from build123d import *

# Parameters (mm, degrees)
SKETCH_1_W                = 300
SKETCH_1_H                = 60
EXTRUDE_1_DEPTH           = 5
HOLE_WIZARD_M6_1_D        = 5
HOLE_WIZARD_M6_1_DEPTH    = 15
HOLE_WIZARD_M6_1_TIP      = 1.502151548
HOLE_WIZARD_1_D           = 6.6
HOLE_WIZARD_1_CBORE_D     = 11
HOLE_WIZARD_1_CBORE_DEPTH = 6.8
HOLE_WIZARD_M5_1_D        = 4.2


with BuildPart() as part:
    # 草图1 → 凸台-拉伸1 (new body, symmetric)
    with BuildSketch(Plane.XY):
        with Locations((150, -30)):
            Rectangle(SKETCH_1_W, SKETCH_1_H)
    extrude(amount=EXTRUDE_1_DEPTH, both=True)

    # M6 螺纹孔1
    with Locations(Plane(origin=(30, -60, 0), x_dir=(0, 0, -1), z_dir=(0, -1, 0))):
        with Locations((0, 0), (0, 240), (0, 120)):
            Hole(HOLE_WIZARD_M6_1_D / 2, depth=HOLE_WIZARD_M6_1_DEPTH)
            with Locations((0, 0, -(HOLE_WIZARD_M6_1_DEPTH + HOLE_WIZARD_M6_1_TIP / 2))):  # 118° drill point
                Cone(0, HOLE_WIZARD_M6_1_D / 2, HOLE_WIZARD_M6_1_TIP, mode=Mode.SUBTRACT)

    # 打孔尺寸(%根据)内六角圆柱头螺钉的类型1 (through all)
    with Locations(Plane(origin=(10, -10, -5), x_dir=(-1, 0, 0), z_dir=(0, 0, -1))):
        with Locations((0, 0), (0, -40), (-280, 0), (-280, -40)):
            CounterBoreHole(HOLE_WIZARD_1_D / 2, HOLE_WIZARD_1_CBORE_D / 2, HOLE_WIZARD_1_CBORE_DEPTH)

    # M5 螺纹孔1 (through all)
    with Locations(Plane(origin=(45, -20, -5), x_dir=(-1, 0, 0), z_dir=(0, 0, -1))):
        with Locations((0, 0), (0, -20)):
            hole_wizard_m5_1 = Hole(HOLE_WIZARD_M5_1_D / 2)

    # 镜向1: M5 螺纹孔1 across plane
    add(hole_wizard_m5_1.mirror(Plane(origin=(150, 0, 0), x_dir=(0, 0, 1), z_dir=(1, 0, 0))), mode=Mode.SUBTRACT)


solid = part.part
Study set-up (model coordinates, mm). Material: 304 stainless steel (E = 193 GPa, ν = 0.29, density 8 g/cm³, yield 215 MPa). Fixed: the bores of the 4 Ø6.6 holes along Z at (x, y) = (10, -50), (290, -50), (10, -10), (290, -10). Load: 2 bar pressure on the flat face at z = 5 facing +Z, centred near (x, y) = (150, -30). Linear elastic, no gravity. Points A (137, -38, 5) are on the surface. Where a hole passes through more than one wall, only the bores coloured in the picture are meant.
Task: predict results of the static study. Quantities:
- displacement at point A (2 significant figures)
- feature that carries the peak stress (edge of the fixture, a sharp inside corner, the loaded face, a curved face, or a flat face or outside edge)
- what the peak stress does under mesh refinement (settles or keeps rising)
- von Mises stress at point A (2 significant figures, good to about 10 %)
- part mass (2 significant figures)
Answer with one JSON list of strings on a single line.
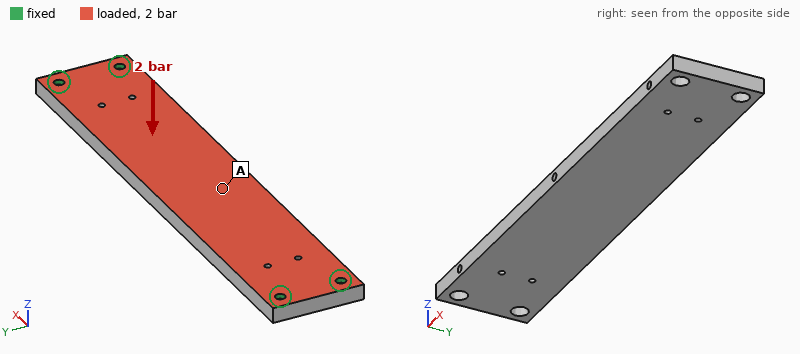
["0.31 mm", "edge of the fixture", "keeps rising", "40 MPa", "1.4 kg"]
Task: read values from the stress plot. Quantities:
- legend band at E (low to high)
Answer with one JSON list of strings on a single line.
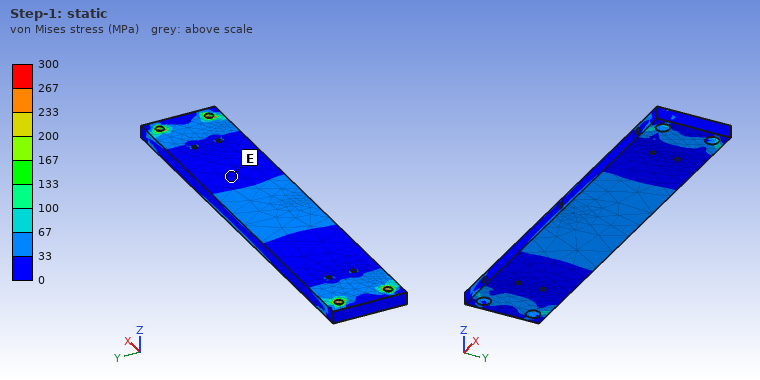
["0 to 33 MPa"]
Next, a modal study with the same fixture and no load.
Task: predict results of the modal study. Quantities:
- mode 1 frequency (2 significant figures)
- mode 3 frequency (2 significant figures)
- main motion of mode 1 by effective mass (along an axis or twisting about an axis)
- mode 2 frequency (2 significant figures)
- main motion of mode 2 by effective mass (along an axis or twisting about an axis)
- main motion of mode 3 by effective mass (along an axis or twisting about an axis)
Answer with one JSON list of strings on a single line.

["510 Hz", "1800 Hz", "along Z", "1400 Hz", "twisting about Y", "twisting about X"]
